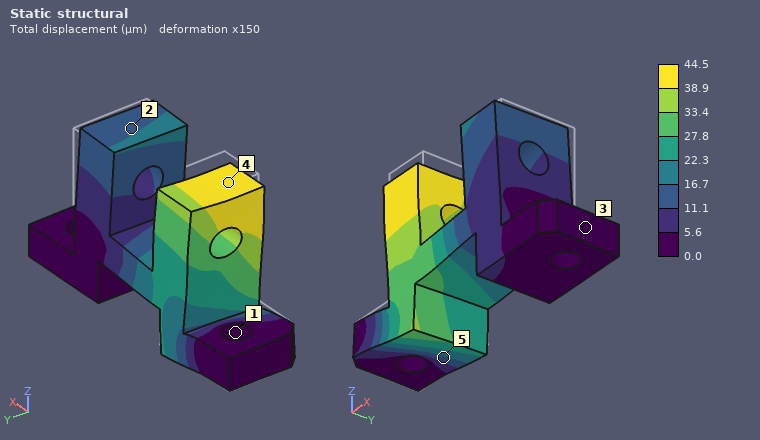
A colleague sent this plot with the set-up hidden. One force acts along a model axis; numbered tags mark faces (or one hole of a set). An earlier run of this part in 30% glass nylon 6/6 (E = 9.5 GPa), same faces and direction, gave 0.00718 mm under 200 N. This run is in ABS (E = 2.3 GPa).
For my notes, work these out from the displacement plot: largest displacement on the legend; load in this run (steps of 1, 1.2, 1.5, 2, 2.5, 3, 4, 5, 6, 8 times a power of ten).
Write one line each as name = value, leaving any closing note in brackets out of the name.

largest displacement on the legend = 44.5 µm
load in this run = 300 N
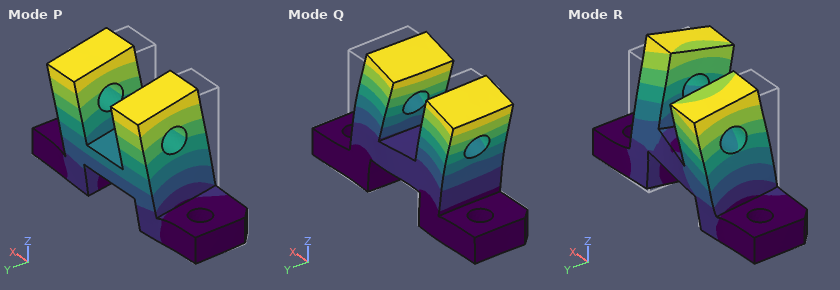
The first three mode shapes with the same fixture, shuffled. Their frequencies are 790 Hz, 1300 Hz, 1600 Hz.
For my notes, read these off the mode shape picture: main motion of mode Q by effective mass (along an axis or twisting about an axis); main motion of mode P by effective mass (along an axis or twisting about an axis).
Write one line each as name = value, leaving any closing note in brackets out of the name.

main motion of mode Q by effective mass = along X
main motion of mode P by effective mass = along Y
